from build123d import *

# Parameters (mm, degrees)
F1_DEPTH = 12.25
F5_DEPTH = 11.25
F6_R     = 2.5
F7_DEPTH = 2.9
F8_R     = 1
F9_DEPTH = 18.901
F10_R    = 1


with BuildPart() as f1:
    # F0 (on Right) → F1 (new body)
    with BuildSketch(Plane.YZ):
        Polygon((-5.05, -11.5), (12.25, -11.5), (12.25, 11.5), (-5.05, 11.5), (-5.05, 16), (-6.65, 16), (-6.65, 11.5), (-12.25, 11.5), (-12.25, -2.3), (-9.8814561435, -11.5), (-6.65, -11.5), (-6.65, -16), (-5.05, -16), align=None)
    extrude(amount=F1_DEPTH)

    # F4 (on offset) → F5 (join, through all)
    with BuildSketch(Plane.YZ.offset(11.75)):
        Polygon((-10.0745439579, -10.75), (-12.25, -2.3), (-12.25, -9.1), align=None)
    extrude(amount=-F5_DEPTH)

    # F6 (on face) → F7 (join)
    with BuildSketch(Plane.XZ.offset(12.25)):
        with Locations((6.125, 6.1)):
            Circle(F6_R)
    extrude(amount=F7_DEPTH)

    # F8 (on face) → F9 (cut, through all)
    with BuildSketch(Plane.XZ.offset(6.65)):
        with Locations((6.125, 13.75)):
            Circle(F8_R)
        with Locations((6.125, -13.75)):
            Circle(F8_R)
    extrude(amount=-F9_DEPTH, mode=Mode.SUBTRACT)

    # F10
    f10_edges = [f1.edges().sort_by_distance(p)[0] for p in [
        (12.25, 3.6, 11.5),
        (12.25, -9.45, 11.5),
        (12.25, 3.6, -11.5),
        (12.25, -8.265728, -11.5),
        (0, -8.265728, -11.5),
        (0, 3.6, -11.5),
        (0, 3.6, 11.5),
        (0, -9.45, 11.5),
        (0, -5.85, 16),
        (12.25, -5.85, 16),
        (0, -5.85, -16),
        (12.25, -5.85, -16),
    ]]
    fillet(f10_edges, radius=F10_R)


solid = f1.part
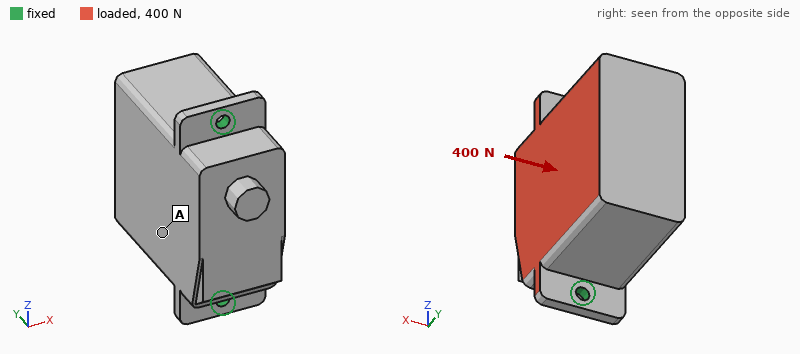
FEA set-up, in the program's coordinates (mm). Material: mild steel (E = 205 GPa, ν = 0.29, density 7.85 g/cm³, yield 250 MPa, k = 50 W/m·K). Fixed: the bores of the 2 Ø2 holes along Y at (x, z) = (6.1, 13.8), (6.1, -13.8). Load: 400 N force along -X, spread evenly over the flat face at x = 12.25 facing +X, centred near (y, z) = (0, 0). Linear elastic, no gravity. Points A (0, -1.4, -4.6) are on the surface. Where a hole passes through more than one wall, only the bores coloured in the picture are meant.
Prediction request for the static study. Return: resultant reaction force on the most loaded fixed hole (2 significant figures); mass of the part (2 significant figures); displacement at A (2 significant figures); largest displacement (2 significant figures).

200 N
55 g
16 µm
39 µm
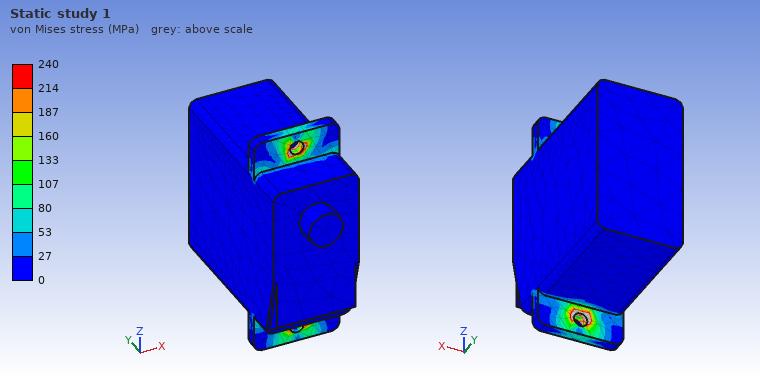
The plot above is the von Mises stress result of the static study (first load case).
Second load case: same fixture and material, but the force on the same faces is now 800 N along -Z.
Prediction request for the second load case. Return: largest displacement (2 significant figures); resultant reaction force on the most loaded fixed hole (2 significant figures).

3.4 µm
480 N
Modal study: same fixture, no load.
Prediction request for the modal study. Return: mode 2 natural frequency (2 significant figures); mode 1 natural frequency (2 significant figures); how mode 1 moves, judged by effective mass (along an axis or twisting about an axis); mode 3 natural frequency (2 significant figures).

12 kHz
2400 Hz
along X
13 kHz
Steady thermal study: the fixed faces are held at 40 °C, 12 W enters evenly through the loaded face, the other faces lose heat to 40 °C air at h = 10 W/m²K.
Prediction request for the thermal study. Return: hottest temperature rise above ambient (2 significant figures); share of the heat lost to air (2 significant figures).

34 K
4.5 %
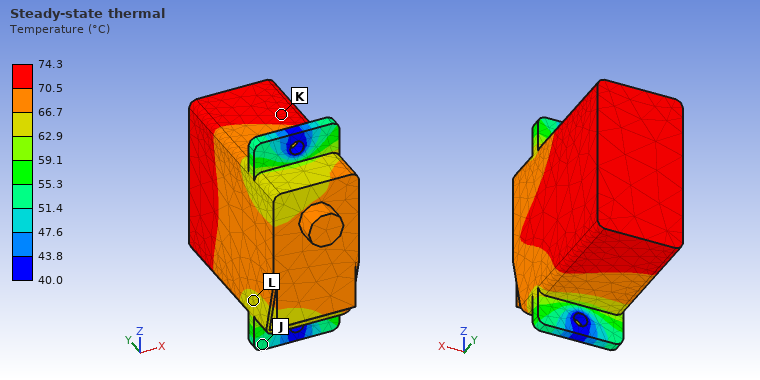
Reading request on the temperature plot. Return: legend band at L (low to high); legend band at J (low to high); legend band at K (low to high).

62.9 to 66.7 °C
51.4 to 55.3 °C
70.5 to 74.3 °C
